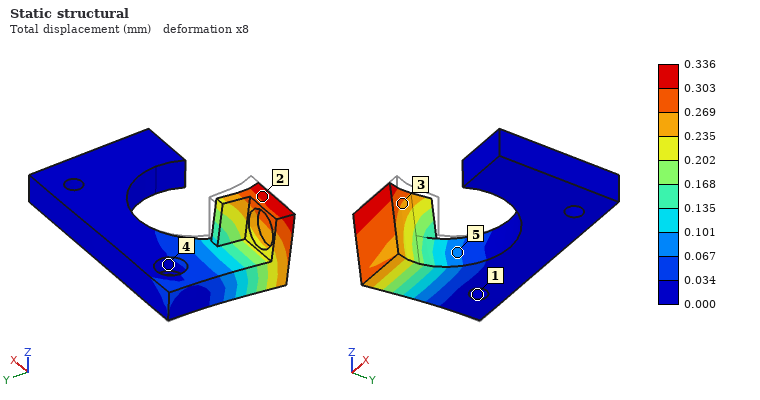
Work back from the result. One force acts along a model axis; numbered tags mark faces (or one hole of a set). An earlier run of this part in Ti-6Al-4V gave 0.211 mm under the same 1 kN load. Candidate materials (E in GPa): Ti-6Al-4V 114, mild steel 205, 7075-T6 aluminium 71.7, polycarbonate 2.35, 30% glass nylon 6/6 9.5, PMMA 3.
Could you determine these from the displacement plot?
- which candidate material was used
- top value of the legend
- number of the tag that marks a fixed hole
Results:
7075-T6 aluminium
0.336 mm
1
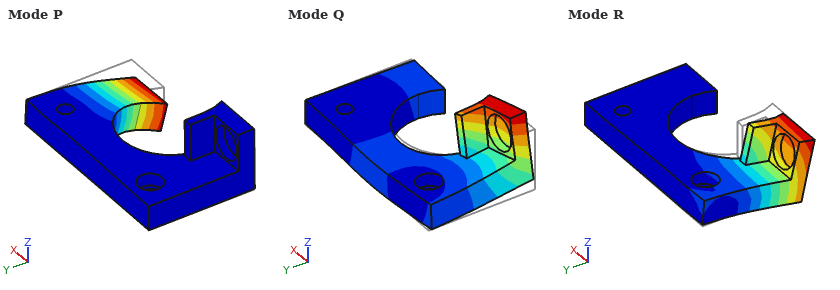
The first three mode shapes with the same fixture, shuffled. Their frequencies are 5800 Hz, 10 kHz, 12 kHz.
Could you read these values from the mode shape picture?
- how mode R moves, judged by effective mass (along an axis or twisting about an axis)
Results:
along Z
